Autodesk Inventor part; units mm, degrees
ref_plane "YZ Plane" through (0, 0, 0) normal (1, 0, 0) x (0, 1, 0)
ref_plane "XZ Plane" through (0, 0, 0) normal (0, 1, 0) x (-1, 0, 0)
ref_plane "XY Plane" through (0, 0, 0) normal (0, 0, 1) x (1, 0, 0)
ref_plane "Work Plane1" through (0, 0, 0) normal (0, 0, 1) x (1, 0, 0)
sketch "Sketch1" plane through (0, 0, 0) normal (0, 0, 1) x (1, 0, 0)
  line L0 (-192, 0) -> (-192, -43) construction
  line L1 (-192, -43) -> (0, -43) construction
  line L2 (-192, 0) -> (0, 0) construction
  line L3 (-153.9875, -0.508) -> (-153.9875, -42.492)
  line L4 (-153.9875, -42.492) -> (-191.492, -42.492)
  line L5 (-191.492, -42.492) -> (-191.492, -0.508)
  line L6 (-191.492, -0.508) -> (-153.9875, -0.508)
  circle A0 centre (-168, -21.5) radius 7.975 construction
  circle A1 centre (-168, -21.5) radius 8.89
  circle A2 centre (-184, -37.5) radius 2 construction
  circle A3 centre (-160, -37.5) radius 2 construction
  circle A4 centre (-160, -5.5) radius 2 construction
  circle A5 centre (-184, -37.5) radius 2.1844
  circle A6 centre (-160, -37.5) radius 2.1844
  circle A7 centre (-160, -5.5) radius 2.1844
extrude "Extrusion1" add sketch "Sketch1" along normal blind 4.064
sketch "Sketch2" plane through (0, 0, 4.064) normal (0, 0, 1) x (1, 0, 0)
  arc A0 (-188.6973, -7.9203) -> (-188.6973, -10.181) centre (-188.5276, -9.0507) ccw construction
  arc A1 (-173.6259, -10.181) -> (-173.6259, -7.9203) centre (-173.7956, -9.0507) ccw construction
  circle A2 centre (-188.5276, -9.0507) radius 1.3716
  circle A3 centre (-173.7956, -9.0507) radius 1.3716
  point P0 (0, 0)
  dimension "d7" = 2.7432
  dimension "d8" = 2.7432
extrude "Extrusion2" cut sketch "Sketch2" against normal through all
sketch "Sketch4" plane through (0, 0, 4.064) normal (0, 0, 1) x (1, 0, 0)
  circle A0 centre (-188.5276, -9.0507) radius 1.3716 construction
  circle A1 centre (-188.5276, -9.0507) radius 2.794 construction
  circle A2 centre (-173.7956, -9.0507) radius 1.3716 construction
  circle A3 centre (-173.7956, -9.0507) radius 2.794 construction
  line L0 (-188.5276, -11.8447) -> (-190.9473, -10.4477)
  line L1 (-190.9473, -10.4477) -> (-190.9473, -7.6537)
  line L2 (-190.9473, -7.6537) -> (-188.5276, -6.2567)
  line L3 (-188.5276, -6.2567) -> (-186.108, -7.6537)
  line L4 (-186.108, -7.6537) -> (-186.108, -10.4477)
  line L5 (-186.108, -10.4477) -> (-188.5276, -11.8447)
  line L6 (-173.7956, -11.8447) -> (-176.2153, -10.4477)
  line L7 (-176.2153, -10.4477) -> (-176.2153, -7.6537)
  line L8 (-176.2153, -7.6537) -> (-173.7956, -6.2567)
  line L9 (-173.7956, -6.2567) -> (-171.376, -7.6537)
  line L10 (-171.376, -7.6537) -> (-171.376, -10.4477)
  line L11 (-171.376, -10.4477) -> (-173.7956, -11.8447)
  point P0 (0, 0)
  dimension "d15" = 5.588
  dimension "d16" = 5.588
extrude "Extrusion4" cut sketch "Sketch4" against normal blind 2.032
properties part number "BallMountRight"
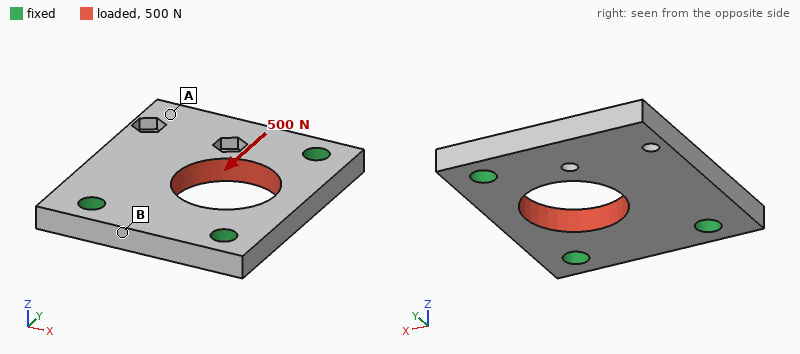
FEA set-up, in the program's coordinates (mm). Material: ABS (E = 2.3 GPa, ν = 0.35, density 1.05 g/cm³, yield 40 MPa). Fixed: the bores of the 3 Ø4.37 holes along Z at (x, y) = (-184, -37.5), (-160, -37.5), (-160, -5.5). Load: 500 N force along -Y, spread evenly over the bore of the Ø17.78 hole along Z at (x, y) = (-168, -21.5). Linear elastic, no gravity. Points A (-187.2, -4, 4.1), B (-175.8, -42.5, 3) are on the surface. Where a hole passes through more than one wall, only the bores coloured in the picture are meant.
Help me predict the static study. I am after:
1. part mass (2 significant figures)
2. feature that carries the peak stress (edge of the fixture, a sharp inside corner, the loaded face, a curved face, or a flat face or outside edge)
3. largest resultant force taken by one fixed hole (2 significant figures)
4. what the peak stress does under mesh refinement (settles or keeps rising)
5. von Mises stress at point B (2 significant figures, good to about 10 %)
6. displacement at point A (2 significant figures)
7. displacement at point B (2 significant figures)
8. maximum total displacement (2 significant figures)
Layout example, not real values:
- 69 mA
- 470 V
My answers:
- 5.4 g
- edge of the fixture
- 180 N
- keeps rising
- 1.9 MPa
- 23 µm
- 15 µm
- 39 µm
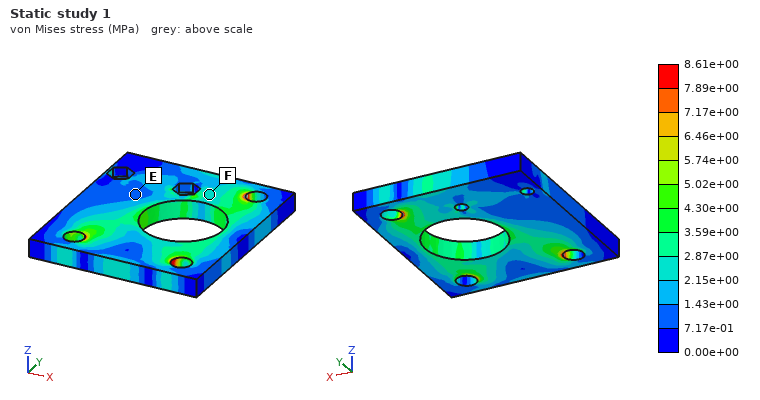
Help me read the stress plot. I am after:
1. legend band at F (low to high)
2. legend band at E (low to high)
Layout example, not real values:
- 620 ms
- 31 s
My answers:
- 2.15e+00 to 2.87e+00 MPa
- 7.17e-01 to 1.43e+00 MPa
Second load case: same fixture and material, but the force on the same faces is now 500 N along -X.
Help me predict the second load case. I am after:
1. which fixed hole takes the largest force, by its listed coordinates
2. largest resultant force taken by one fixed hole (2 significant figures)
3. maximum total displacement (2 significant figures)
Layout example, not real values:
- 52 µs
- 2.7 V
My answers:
- (-160, -5.5)
- 230 N
- 68 µm
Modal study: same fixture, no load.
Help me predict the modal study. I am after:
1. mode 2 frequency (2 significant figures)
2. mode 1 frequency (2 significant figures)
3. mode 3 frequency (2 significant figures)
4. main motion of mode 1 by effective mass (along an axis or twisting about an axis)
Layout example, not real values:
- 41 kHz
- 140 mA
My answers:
- 4700 Hz
- 1600 Hz
- 5900 Hz
- along Z
